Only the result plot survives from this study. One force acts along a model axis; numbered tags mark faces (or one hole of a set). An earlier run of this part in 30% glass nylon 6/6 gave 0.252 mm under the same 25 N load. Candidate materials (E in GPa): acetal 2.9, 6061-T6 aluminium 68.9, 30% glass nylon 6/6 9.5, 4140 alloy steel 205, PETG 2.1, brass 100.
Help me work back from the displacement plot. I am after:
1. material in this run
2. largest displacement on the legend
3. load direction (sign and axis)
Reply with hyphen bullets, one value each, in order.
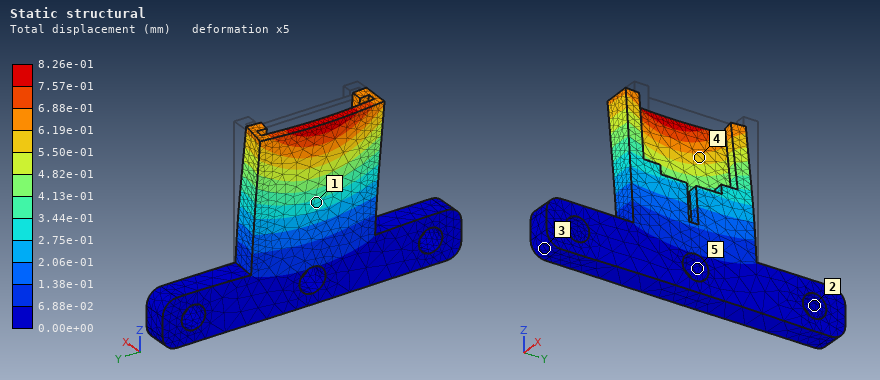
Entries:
- acetal
- 8.26e-01 mm
- -X
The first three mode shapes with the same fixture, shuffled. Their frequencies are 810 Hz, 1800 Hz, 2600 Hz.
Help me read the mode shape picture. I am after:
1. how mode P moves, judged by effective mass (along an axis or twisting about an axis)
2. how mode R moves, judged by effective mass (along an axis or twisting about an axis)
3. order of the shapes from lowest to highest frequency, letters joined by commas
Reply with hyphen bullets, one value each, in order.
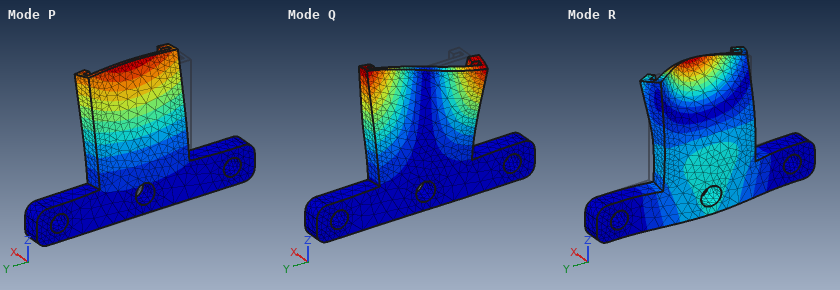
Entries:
- along X
- along X
- P, Q, R
